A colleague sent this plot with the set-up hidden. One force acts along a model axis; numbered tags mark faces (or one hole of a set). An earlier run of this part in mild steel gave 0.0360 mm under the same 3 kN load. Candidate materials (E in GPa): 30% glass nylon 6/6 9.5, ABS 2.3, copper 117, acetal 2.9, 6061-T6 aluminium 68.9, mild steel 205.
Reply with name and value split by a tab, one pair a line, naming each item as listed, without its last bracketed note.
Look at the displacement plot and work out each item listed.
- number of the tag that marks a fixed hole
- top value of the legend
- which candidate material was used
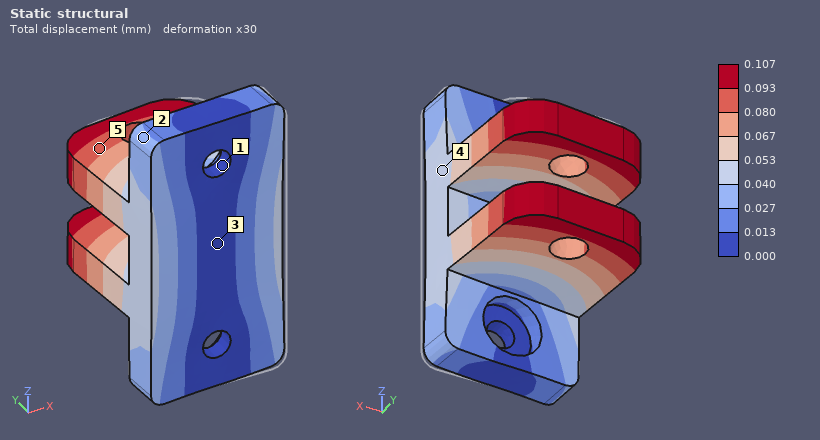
number of the tag that marks a fixed hole	1
top value of the legend	0.107 mm
which candidate material was used	6061-T6 aluminium
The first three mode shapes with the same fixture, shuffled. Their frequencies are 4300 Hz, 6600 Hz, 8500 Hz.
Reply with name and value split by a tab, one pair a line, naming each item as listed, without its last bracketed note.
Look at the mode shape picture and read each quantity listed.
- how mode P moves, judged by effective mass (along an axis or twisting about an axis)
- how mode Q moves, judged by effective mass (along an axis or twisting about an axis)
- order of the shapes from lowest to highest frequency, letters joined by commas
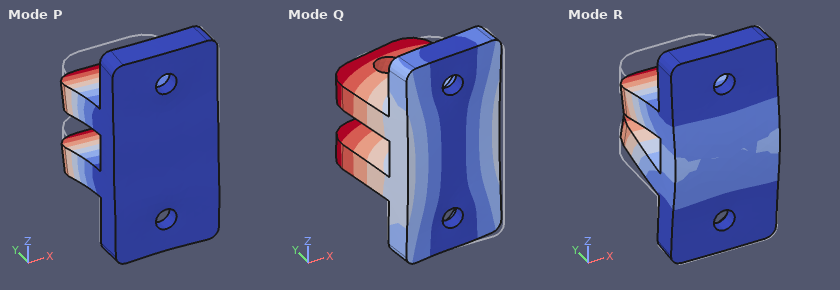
how mode P moves, judged by effective mass	along Z
how mode Q moves, judged by effective mass	along X
order of the shapes from lowest to highest frequency, letters joined by commas	Q, R, P
